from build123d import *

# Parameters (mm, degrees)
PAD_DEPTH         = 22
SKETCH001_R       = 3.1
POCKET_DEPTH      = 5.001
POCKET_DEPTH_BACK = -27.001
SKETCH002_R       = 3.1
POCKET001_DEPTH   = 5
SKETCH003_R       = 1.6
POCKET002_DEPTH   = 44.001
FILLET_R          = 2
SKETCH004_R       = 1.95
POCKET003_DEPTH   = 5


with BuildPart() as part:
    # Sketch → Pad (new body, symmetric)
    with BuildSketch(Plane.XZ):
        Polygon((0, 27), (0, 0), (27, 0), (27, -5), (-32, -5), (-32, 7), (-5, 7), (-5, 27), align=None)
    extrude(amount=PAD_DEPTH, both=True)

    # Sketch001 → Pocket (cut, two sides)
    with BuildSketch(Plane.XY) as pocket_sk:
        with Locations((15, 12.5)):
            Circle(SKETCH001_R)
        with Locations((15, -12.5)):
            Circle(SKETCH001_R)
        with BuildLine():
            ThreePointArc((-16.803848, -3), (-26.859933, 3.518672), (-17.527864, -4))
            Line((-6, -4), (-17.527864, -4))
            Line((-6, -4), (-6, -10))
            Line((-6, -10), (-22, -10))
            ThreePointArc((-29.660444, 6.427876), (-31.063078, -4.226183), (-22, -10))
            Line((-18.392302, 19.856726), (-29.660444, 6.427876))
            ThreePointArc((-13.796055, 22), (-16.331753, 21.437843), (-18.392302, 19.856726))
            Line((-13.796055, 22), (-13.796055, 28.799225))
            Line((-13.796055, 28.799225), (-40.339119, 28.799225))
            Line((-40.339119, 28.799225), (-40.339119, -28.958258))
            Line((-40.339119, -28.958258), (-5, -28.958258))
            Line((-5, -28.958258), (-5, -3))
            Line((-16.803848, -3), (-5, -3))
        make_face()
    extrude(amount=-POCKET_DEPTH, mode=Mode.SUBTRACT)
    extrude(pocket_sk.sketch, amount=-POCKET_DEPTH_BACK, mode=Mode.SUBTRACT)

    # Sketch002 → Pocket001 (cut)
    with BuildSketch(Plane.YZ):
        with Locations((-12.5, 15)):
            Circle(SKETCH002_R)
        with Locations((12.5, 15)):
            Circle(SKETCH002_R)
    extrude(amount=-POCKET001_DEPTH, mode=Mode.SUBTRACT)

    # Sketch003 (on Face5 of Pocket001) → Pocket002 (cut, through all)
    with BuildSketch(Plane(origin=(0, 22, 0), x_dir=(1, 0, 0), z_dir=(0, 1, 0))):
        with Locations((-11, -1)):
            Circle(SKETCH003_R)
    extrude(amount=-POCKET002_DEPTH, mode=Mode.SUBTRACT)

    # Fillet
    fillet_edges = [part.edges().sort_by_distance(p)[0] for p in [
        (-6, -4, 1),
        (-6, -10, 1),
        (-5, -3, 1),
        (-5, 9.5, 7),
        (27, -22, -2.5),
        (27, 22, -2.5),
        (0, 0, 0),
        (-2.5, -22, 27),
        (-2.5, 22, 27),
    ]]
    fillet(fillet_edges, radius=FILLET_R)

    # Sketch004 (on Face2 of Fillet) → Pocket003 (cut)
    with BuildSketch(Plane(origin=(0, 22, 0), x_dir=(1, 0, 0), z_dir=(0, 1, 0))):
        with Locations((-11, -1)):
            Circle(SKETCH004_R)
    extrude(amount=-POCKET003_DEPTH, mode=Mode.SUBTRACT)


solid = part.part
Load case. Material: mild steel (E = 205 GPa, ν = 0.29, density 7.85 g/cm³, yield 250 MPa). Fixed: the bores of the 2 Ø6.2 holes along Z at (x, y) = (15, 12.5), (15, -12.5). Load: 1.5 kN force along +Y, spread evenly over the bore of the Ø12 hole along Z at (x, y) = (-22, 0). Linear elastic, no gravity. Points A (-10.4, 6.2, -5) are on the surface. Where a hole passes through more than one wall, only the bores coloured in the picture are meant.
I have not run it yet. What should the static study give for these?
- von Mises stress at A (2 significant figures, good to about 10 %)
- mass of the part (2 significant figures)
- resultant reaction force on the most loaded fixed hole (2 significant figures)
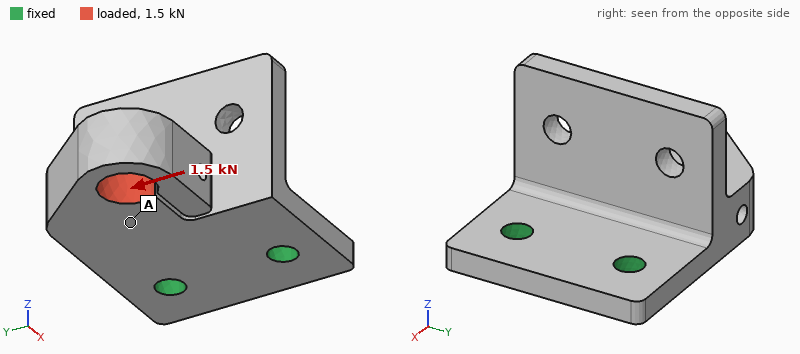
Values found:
20 MPa
150 g
2.2 kN
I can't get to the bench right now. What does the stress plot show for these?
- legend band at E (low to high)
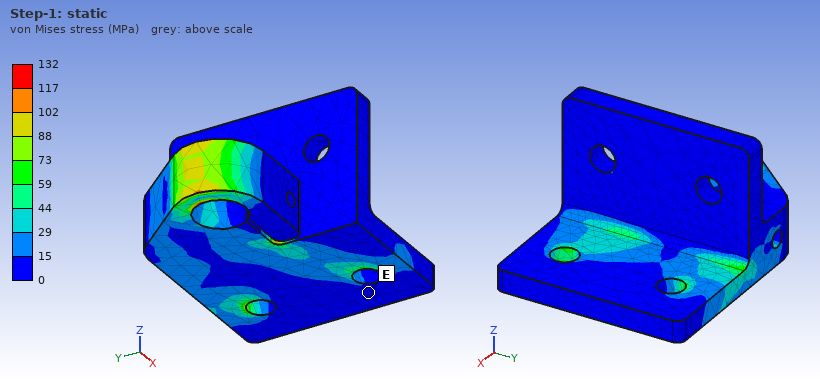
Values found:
0 to 15 MPa
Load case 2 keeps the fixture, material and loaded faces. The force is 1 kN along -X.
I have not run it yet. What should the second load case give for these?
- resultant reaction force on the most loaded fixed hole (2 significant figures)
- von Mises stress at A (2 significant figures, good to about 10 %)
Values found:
530 N
9.6 MPa
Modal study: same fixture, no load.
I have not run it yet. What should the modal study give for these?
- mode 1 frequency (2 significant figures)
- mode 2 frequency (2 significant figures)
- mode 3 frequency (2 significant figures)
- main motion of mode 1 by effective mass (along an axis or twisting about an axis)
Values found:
1700 Hz
2500 Hz
3300 Hz
along Z
